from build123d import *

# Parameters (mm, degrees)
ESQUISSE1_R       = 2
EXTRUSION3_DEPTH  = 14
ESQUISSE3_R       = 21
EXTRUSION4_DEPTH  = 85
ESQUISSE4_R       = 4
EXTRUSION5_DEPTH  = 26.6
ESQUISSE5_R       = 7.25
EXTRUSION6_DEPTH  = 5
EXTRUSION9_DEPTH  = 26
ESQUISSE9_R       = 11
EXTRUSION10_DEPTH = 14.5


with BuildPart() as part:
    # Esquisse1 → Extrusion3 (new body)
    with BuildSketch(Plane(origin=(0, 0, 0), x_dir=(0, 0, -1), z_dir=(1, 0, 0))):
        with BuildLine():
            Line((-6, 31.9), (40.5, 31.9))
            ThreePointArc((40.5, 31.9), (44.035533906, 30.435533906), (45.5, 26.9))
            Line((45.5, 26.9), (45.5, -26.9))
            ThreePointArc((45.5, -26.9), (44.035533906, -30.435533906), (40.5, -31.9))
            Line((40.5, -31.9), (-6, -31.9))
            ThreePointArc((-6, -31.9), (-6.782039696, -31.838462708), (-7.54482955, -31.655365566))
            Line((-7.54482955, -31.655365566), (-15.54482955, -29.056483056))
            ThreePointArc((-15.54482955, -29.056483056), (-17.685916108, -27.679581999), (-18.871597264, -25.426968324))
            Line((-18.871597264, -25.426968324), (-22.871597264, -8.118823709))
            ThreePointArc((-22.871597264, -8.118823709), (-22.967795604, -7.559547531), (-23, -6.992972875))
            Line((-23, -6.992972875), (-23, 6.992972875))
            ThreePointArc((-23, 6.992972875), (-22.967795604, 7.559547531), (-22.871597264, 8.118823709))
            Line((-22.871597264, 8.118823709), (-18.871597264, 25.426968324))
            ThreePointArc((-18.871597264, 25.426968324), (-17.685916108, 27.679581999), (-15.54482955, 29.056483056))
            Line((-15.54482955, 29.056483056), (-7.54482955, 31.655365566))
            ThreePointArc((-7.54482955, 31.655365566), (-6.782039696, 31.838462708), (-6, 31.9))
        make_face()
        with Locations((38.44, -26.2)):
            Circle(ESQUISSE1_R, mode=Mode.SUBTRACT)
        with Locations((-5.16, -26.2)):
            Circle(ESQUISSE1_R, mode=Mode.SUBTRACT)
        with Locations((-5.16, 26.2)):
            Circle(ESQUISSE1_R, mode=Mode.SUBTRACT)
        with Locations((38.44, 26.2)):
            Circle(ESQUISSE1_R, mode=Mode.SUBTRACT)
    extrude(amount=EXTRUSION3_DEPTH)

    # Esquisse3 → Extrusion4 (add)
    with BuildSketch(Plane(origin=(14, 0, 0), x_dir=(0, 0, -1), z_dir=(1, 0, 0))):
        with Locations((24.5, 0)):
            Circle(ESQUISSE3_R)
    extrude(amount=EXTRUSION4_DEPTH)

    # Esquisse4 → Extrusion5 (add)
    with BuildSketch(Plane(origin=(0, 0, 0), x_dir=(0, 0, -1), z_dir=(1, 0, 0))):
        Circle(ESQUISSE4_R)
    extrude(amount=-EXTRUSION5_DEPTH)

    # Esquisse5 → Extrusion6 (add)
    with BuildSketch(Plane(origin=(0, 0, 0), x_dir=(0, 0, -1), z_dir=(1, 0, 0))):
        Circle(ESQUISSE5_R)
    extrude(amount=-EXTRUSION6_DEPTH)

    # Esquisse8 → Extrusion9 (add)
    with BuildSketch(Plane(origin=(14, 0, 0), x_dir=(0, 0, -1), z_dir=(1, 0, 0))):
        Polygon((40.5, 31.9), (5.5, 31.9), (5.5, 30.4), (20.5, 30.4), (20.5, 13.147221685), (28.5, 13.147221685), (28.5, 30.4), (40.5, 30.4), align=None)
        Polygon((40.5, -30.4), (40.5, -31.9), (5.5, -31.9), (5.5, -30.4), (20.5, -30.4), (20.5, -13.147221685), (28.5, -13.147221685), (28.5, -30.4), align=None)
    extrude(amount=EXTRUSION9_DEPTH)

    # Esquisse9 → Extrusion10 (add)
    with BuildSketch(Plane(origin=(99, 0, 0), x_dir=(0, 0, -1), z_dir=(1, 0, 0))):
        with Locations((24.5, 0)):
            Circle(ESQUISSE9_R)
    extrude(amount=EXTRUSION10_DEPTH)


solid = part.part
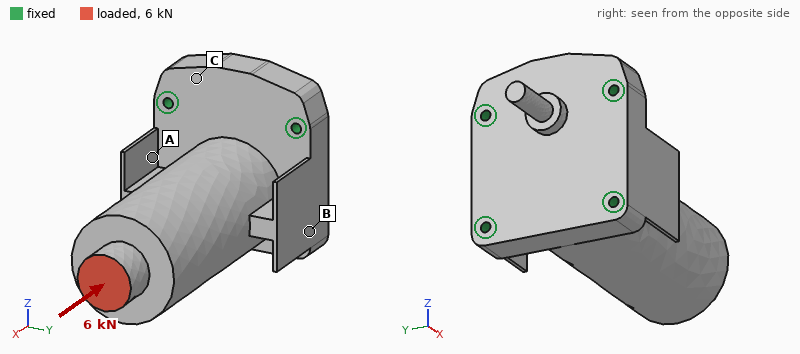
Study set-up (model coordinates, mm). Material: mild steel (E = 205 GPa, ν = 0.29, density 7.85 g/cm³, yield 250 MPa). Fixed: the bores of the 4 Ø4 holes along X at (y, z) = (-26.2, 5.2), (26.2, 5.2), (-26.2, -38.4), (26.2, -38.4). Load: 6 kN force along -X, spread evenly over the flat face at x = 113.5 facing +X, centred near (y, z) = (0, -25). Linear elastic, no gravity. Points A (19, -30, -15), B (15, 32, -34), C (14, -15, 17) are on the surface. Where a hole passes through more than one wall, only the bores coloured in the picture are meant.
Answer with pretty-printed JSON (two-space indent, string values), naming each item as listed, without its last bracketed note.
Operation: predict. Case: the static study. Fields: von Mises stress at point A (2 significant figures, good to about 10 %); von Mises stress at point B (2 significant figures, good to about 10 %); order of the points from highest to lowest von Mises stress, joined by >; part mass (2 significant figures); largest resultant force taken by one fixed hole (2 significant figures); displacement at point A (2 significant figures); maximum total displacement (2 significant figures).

{
  "von Mises stress at point A": "6.8 MPa",
  "von Mises stress at point B": "12 MPa",
  "order of the points from highest to lowest von Mises stress, joined by >": "B > A > C",
  "part mass": "1.5 kg",
  "largest resultant force taken by one fixed hole": "2.1 kN",
  "displacement at point A": "1.2 µm",
  "maximum total displacement": "5.0 µm"
}
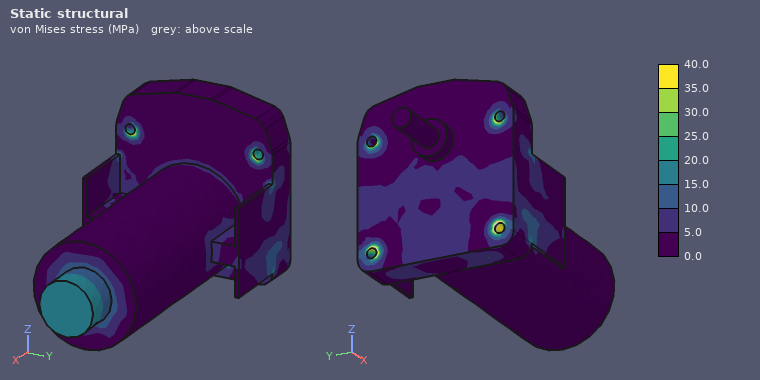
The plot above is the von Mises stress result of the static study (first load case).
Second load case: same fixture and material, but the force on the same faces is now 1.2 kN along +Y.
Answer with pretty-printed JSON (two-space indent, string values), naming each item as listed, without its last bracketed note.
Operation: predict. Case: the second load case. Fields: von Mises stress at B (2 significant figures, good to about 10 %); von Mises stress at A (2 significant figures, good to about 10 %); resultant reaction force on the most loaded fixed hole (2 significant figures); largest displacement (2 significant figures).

{
  "von Mises stress at B": "17 MPa",
  "von Mises stress at A": "9.2 MPa",
  "resultant reaction force on the most loaded fixed hole": "1.9 kN",
  "largest displacement": "19 µm"
}
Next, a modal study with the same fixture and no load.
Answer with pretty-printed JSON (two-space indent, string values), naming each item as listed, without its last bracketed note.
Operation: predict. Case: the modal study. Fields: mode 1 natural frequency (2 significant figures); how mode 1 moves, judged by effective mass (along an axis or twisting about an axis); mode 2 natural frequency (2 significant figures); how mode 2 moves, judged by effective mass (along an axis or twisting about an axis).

{
  "mode 1 natural frequency": "2200 Hz",
  "how mode 1 moves, judged by effective mass": "along Z",
  "mode 2 natural frequency": "2800 Hz",
  "how mode 2 moves, judged by effective mass": "along Y"
}
